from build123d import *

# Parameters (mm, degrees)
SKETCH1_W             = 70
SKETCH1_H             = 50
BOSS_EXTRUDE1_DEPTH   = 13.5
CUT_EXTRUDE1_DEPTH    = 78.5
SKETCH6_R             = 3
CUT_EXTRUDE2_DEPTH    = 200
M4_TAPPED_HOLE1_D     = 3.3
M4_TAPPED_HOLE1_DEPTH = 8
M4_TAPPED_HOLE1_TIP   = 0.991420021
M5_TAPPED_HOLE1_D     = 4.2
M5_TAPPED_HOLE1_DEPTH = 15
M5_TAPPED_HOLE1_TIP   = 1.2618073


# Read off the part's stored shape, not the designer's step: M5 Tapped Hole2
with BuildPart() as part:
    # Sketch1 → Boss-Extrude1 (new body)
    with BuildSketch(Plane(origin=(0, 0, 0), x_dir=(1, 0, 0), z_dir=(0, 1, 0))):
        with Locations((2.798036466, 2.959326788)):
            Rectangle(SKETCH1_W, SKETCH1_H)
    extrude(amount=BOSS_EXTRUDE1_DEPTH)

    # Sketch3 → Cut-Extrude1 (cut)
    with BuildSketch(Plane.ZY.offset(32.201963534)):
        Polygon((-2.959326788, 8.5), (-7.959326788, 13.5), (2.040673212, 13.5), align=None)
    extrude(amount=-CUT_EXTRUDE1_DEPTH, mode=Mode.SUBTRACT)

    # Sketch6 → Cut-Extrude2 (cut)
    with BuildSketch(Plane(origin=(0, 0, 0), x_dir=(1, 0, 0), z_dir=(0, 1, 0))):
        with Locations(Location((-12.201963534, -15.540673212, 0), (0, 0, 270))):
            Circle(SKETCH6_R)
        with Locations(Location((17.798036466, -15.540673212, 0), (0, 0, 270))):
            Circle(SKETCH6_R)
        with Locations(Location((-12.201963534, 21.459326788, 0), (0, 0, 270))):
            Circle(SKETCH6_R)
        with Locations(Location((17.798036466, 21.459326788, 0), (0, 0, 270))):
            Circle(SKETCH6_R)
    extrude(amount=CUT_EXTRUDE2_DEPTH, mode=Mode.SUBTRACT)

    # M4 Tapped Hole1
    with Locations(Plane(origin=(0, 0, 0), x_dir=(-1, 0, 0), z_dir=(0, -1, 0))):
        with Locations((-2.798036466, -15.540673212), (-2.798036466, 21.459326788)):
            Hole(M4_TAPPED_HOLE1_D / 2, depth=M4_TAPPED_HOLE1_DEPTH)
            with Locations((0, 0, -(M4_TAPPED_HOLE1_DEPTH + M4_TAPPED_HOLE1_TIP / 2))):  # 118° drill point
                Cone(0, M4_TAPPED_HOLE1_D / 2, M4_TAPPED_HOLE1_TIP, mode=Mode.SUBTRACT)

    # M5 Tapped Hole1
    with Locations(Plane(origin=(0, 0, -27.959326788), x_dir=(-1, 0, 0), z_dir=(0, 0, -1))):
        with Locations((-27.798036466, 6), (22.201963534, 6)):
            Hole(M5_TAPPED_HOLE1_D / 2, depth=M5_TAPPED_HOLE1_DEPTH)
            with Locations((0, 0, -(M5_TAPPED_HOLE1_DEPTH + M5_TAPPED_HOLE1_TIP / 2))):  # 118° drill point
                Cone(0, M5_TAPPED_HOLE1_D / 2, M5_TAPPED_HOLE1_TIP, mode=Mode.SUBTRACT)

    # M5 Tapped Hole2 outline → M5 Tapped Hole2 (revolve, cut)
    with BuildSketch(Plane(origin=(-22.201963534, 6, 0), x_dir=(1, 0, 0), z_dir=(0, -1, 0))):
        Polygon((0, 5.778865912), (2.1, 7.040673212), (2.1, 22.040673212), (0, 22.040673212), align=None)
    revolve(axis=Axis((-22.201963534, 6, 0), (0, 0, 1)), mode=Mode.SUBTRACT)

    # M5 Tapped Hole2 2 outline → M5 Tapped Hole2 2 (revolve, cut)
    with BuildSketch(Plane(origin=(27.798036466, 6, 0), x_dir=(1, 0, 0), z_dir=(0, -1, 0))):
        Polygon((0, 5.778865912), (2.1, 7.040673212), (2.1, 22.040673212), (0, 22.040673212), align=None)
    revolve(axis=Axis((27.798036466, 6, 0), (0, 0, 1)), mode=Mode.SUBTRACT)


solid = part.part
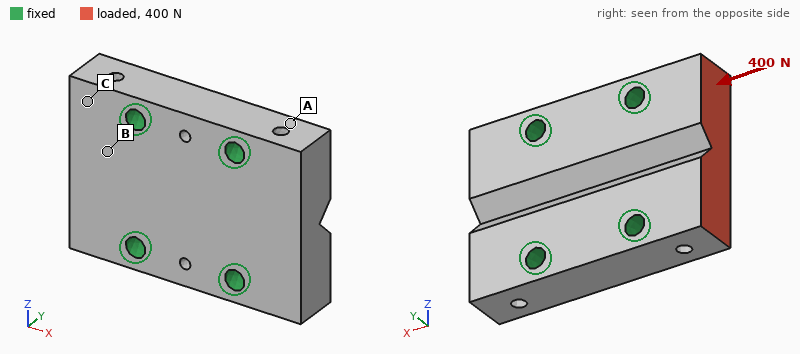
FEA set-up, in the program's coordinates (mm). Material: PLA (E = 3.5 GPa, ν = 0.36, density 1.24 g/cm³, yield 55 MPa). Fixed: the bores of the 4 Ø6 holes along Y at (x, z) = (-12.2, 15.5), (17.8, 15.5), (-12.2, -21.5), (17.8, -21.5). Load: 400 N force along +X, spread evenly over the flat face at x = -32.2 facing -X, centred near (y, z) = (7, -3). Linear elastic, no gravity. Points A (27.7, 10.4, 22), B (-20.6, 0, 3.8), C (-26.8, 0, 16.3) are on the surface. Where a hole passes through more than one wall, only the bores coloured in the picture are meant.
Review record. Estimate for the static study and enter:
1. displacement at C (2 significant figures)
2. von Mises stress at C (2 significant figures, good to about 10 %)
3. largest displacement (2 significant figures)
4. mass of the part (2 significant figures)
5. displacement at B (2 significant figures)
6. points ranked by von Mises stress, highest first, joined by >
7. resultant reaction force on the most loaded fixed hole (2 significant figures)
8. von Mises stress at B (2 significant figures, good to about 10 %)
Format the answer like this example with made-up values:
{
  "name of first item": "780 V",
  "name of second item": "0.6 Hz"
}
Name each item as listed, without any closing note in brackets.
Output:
{
  "displacement at C": "3.4 µm",
  "von Mises stress at C": "0.82 MPa",
  "largest displacement": "5.3 µm",
  "mass of the part": "53 g",
  "displacement at B": "3.3 µm",
  "points ranked by von Mises stress, highest first, joined by >": "C > B > A",
  "resultant reaction force on the most loaded fixed hole": "170 N",
  "von Mises stress at B": "0.48 MPa"
}
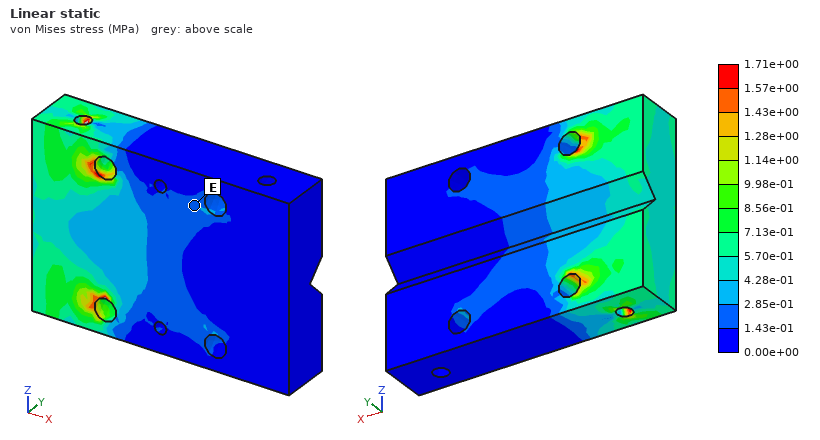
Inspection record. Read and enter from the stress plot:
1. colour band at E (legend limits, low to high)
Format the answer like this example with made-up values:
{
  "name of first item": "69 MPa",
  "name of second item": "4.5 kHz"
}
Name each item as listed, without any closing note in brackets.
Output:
{
  "colour band at E": "1.43e-01 to 2.85e-01 MPa"
}
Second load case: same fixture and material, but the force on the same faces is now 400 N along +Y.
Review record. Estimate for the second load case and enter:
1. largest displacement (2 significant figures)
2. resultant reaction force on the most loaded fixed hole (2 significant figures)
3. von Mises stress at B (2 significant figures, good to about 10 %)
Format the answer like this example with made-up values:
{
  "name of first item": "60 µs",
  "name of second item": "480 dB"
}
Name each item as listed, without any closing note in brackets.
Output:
{
  "largest displacement": "60 µm",
  "resultant reaction force on the most loaded fixed hole": "230 N",
  "von Mises stress at B": "2.4 MPa"
}
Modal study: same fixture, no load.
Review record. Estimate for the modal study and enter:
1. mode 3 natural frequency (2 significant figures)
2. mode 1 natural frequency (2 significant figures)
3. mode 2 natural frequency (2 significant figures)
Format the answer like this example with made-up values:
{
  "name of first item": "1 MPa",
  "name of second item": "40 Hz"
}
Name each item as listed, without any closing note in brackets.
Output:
{
  "mode 3 natural frequency": "8400 Hz",
  "mode 1 natural frequency": "6000 Hz",
  "mode 2 natural frequency": "6100 Hz"
}
